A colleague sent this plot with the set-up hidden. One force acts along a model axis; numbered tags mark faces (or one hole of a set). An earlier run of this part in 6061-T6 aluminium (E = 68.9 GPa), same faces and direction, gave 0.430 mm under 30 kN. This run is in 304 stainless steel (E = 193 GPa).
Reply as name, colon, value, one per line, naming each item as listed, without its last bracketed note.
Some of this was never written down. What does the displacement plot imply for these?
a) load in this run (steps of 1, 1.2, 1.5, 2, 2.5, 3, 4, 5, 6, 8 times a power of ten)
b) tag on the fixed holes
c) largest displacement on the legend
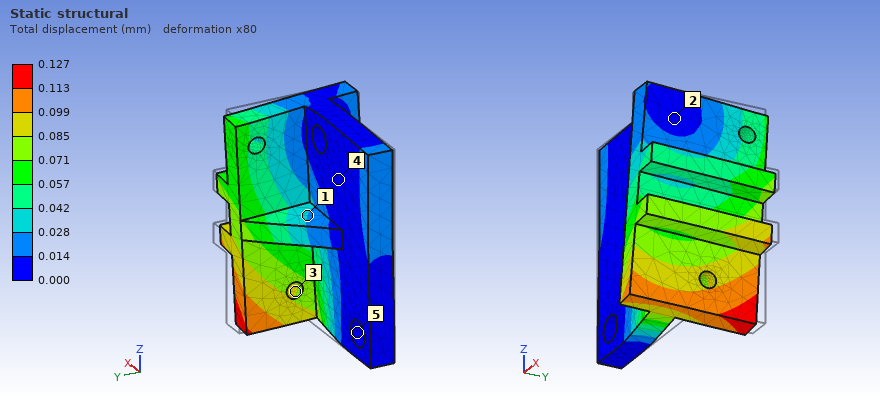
load in this run: 25 kN
tag on the fixed holes: 5
largest displacement on the legend: 0.127 mm
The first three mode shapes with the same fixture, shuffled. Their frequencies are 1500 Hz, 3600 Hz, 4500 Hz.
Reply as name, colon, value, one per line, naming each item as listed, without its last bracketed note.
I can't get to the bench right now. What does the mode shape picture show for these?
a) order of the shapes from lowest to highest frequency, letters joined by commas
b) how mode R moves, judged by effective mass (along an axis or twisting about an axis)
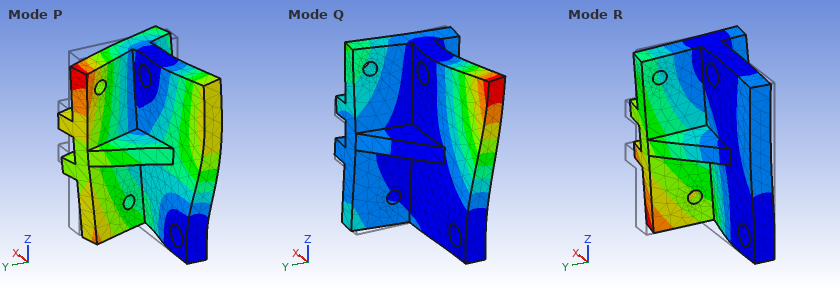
order of the shapes from lowest to highest frequency, letters joined by commas: R, P, Q
how mode R moves, judged by effective mass: along Y
